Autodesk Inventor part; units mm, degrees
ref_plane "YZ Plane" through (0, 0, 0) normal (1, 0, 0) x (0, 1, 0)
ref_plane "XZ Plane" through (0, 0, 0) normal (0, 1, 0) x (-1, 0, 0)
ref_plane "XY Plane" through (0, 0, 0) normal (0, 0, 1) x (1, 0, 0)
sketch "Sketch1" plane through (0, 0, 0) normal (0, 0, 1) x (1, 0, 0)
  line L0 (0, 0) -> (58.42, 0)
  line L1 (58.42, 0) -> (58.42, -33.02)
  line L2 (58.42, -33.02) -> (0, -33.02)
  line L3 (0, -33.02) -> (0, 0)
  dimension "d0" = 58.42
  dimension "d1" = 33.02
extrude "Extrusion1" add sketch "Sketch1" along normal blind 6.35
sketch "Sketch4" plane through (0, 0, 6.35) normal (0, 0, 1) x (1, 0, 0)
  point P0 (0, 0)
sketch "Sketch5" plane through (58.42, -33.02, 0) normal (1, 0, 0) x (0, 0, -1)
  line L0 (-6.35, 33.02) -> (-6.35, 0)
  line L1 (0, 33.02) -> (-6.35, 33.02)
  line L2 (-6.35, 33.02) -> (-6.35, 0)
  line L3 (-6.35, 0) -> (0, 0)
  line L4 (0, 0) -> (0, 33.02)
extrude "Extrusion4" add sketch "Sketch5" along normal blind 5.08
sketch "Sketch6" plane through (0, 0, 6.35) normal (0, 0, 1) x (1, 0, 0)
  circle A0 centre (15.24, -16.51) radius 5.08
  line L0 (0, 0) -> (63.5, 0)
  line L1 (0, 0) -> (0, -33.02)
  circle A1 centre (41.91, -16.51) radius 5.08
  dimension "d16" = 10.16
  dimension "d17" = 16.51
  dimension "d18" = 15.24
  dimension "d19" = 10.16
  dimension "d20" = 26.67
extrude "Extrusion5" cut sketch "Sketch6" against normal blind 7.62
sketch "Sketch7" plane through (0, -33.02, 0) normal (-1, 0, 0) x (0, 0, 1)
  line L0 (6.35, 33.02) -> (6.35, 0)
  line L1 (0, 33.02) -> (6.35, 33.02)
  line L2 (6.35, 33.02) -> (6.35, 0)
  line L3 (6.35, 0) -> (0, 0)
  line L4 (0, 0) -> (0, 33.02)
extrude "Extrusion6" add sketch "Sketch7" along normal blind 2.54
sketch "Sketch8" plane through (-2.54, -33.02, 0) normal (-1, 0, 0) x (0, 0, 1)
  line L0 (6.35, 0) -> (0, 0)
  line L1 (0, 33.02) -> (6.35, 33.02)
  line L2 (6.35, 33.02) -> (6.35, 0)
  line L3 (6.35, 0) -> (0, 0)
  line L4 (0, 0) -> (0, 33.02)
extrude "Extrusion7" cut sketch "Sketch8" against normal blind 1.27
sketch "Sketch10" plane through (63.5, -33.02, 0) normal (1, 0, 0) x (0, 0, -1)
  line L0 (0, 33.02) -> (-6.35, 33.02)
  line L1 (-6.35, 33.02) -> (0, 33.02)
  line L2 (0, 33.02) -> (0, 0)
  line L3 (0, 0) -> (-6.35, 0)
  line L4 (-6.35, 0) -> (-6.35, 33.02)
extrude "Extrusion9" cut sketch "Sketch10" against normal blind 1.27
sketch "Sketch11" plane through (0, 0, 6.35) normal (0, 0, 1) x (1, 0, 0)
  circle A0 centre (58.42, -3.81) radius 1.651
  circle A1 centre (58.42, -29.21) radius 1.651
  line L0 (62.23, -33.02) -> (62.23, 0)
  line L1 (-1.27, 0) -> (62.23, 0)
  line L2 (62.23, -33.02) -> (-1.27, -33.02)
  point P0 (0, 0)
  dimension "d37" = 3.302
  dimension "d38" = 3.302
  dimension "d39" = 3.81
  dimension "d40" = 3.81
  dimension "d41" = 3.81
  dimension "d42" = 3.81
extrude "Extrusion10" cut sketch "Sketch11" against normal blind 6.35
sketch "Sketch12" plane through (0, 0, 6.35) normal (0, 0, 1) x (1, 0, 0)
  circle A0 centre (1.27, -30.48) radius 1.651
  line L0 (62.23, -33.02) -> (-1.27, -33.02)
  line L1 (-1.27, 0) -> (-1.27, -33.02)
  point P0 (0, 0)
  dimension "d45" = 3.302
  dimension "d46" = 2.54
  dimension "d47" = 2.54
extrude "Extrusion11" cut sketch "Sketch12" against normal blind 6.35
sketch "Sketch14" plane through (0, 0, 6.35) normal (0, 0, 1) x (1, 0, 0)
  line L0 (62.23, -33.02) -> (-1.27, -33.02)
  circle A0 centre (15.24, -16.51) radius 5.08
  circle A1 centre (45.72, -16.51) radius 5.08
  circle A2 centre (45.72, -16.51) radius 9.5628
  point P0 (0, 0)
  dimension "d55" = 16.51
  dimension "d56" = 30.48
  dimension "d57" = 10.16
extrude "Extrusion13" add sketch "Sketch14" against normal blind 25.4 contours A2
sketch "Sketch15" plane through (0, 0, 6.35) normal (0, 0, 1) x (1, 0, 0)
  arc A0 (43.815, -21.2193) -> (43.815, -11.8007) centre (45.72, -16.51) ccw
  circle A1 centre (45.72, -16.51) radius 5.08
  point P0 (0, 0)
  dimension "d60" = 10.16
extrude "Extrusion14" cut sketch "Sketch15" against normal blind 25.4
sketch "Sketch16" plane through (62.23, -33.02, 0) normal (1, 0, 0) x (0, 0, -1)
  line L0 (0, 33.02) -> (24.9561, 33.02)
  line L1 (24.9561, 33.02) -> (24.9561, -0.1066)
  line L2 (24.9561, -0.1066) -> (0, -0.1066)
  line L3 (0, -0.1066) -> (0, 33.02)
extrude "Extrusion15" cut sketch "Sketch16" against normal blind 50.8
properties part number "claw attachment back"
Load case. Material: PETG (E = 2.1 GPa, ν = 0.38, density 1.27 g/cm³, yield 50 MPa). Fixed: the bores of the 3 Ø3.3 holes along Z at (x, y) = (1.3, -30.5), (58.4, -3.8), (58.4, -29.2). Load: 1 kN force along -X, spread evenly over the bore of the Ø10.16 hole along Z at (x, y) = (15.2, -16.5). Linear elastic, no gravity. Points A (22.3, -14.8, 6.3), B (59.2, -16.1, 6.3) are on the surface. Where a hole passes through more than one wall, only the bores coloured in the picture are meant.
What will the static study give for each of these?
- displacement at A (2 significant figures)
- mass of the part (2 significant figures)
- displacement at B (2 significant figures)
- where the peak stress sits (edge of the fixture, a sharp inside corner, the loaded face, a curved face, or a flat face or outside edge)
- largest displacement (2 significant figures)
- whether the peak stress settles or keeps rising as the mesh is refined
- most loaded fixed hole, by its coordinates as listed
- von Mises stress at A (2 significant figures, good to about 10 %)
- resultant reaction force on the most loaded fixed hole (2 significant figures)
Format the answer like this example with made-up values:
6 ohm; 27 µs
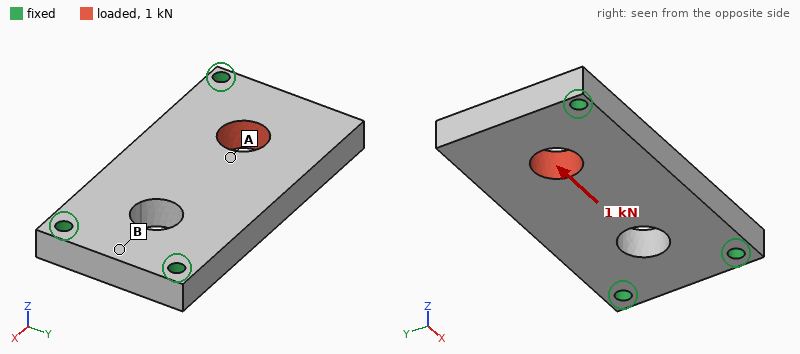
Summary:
0.080 mm; 15 g; 0.019 mm; edge of the fixture; 0.11 mm; keeps rising; (1.3, -30.5); 5.9 MPa; 420 N
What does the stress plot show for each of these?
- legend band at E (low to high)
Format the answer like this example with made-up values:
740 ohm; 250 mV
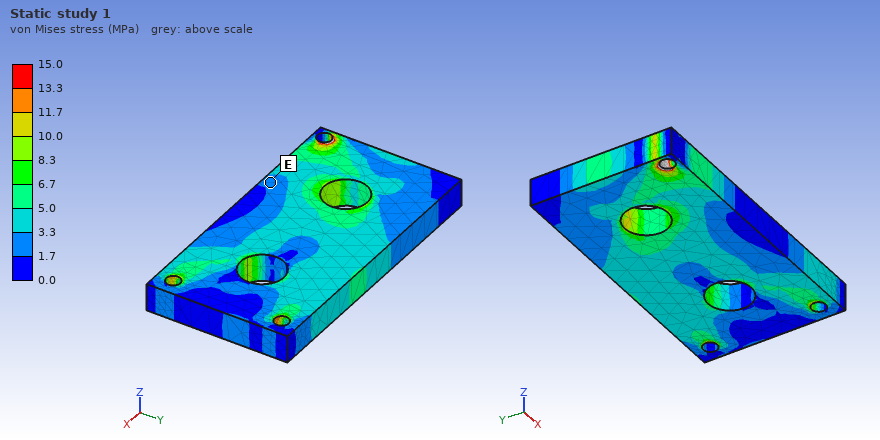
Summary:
1.7 to 3.3 MPa
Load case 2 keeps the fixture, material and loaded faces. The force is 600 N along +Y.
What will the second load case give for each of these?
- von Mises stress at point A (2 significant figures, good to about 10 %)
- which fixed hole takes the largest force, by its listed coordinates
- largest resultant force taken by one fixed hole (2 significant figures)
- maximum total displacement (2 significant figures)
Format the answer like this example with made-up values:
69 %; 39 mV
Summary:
1.9 MPa; (1.3, -30.5); 440 N; 98 µm
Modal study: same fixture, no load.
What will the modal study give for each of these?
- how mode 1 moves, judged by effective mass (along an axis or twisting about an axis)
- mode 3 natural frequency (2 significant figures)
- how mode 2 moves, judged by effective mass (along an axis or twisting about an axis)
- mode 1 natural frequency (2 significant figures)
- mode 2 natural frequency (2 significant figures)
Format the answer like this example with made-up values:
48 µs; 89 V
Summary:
along Z; 3500 Hz; along Z; 1200 Hz; 2300 Hz
